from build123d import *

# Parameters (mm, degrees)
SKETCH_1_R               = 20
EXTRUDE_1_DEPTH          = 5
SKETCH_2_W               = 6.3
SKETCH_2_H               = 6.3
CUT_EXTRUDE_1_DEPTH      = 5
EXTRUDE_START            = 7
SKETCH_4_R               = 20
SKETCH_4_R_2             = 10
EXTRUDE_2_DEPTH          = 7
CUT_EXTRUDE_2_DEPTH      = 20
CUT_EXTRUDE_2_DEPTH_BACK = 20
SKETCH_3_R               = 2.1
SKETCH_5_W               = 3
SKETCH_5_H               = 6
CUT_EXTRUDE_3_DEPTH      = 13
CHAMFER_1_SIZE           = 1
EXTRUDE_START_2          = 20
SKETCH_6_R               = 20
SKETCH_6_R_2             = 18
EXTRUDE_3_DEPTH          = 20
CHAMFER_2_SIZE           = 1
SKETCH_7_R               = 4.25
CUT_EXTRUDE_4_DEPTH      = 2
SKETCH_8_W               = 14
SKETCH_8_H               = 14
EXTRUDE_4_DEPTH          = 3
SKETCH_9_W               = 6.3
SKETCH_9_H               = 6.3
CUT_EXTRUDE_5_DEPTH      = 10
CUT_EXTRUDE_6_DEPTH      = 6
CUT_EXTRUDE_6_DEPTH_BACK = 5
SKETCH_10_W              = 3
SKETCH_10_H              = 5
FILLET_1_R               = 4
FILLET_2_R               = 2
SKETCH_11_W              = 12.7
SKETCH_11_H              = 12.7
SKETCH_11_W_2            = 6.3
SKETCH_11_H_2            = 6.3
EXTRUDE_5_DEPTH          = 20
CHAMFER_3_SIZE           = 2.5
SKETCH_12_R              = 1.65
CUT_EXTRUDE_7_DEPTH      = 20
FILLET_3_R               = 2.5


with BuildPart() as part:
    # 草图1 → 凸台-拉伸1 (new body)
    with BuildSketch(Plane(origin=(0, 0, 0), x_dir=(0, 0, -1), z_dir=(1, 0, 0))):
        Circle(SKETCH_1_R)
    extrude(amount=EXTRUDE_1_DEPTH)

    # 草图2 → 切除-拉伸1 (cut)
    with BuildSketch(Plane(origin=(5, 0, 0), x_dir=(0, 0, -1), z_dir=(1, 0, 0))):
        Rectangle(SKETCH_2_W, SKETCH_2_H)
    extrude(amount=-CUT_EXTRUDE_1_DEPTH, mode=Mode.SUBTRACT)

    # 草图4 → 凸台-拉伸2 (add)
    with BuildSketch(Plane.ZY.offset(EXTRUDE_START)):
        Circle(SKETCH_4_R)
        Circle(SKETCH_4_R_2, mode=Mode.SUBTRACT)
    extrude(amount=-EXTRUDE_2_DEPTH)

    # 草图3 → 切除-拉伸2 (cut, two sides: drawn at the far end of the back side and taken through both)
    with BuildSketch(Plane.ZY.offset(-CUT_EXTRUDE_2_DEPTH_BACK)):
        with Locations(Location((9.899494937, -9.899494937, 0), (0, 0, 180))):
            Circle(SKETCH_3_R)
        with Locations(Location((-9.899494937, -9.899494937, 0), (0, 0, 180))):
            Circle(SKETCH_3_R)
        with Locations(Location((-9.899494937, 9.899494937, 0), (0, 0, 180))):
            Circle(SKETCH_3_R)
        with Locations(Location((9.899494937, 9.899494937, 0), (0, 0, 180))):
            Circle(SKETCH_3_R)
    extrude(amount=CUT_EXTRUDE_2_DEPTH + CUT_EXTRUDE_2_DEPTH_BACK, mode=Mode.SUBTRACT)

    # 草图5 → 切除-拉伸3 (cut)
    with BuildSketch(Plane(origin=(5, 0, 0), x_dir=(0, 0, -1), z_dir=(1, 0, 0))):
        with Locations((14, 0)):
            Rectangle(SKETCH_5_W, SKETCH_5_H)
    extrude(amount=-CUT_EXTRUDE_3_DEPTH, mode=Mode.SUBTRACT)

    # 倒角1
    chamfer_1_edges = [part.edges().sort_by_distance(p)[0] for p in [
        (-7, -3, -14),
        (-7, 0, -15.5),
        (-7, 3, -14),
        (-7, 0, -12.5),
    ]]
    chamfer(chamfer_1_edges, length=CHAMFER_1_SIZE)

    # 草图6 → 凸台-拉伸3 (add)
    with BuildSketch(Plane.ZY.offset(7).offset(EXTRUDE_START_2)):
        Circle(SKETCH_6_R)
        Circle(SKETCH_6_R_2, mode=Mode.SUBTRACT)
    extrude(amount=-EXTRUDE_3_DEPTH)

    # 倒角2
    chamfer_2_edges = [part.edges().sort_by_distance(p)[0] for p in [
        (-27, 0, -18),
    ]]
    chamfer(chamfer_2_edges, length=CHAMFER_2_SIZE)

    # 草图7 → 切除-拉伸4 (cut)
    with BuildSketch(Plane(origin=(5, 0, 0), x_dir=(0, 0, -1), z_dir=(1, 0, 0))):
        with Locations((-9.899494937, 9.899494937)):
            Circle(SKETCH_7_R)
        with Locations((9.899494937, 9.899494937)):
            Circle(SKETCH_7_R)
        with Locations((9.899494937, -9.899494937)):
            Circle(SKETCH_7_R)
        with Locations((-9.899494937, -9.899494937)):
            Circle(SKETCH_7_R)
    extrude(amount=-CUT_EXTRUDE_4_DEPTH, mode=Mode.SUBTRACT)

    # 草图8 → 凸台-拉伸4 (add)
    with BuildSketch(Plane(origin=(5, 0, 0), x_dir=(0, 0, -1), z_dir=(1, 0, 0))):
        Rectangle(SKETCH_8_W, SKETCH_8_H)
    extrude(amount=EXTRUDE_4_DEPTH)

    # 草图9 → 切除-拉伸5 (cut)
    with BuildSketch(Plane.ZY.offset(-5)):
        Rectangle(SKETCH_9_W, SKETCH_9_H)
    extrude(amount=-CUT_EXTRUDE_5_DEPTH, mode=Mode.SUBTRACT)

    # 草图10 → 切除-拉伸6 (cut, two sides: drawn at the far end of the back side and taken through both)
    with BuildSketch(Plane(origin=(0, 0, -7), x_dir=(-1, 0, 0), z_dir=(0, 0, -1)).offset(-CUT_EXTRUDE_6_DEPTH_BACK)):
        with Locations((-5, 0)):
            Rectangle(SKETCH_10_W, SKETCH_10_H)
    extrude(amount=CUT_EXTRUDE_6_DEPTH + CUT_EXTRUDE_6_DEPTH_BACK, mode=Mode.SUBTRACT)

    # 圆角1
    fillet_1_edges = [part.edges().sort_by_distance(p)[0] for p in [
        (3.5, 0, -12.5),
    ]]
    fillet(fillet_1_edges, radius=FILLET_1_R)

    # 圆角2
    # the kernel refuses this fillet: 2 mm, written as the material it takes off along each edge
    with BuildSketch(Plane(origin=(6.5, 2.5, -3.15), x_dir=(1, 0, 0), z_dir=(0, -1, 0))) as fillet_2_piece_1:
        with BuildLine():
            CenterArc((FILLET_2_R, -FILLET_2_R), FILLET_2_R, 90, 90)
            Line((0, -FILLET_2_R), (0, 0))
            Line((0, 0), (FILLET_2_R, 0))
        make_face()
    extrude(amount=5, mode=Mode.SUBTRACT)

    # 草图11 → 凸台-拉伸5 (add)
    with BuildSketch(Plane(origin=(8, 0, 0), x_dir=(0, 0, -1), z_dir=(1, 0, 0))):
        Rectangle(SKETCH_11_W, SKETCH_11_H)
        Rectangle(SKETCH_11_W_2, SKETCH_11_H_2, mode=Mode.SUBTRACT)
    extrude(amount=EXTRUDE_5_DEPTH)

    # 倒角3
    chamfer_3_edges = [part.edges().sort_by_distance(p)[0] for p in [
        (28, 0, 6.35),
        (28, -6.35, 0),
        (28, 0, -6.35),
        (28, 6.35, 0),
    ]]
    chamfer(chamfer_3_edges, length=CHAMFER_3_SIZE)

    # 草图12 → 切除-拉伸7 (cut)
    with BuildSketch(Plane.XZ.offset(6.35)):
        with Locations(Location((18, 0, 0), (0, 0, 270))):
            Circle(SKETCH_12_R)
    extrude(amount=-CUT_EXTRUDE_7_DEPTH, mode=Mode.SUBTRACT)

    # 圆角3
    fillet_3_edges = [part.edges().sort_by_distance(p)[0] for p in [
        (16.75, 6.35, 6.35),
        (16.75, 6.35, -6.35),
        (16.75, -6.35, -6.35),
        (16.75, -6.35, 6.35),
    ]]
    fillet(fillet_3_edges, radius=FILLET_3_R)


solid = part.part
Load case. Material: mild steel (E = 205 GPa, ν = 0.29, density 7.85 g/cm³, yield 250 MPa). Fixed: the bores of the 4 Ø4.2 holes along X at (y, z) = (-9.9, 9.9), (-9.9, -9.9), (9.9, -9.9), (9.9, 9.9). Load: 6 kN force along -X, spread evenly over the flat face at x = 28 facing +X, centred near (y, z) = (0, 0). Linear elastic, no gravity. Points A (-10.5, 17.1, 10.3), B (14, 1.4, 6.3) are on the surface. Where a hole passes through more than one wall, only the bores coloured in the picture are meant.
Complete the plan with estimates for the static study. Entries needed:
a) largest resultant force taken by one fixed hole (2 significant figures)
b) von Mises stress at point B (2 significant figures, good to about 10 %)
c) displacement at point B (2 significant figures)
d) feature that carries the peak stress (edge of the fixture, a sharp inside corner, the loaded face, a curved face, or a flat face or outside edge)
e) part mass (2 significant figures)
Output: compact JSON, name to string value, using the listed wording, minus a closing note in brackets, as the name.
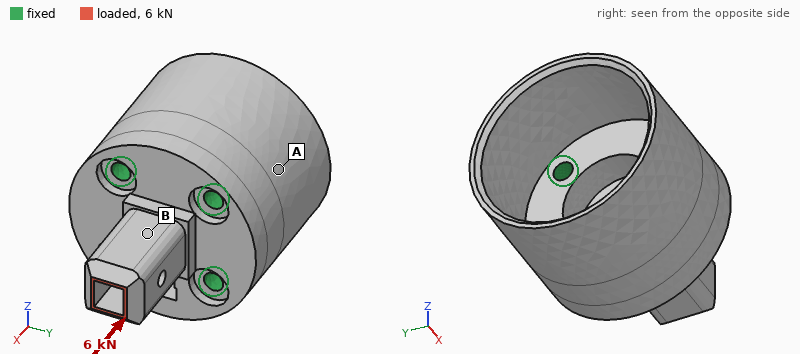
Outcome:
{"largest resultant force taken by one fixed hole": "1.7 kN", "von Mises stress at point B": "53 MPa", "displacement at point B": "5.1 µm", "feature that carries the peak stress": "the loaded face", "part mass": "150 g"}
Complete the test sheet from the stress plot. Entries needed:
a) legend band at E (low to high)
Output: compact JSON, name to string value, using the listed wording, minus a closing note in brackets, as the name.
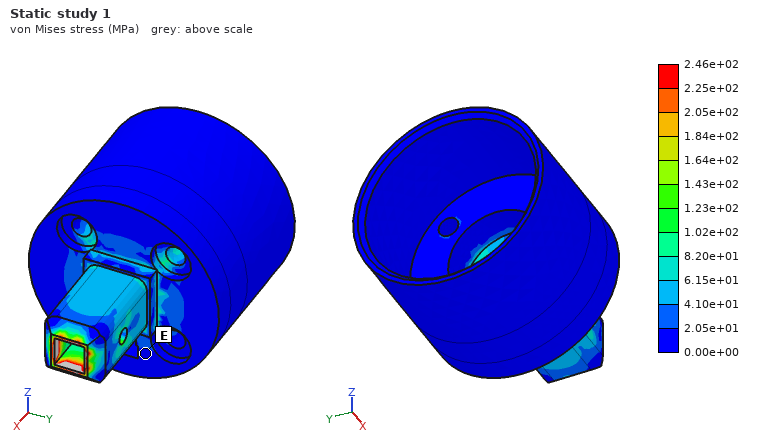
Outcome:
{"legend band at E": "0.00e+00 to 2.05e+01 MPa"}
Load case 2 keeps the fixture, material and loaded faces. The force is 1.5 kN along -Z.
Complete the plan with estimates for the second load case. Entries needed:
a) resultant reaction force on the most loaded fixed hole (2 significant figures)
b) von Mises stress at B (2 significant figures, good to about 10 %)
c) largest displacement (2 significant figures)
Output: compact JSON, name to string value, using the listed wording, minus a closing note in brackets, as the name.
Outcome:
{"resultant reaction force on the most loaded fixed hole": "1.3 kN", "von Mises stress at B": "78 MPa", "largest displacement": "38 µm"}
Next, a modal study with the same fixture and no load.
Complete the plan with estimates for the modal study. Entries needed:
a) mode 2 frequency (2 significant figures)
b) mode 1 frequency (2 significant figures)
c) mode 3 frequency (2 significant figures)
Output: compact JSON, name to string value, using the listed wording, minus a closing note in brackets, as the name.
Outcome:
{"mode 2 frequency": "13 kHz", "mode 1 frequency": "12 kHz", "mode 3 frequency": "14 kHz"}
